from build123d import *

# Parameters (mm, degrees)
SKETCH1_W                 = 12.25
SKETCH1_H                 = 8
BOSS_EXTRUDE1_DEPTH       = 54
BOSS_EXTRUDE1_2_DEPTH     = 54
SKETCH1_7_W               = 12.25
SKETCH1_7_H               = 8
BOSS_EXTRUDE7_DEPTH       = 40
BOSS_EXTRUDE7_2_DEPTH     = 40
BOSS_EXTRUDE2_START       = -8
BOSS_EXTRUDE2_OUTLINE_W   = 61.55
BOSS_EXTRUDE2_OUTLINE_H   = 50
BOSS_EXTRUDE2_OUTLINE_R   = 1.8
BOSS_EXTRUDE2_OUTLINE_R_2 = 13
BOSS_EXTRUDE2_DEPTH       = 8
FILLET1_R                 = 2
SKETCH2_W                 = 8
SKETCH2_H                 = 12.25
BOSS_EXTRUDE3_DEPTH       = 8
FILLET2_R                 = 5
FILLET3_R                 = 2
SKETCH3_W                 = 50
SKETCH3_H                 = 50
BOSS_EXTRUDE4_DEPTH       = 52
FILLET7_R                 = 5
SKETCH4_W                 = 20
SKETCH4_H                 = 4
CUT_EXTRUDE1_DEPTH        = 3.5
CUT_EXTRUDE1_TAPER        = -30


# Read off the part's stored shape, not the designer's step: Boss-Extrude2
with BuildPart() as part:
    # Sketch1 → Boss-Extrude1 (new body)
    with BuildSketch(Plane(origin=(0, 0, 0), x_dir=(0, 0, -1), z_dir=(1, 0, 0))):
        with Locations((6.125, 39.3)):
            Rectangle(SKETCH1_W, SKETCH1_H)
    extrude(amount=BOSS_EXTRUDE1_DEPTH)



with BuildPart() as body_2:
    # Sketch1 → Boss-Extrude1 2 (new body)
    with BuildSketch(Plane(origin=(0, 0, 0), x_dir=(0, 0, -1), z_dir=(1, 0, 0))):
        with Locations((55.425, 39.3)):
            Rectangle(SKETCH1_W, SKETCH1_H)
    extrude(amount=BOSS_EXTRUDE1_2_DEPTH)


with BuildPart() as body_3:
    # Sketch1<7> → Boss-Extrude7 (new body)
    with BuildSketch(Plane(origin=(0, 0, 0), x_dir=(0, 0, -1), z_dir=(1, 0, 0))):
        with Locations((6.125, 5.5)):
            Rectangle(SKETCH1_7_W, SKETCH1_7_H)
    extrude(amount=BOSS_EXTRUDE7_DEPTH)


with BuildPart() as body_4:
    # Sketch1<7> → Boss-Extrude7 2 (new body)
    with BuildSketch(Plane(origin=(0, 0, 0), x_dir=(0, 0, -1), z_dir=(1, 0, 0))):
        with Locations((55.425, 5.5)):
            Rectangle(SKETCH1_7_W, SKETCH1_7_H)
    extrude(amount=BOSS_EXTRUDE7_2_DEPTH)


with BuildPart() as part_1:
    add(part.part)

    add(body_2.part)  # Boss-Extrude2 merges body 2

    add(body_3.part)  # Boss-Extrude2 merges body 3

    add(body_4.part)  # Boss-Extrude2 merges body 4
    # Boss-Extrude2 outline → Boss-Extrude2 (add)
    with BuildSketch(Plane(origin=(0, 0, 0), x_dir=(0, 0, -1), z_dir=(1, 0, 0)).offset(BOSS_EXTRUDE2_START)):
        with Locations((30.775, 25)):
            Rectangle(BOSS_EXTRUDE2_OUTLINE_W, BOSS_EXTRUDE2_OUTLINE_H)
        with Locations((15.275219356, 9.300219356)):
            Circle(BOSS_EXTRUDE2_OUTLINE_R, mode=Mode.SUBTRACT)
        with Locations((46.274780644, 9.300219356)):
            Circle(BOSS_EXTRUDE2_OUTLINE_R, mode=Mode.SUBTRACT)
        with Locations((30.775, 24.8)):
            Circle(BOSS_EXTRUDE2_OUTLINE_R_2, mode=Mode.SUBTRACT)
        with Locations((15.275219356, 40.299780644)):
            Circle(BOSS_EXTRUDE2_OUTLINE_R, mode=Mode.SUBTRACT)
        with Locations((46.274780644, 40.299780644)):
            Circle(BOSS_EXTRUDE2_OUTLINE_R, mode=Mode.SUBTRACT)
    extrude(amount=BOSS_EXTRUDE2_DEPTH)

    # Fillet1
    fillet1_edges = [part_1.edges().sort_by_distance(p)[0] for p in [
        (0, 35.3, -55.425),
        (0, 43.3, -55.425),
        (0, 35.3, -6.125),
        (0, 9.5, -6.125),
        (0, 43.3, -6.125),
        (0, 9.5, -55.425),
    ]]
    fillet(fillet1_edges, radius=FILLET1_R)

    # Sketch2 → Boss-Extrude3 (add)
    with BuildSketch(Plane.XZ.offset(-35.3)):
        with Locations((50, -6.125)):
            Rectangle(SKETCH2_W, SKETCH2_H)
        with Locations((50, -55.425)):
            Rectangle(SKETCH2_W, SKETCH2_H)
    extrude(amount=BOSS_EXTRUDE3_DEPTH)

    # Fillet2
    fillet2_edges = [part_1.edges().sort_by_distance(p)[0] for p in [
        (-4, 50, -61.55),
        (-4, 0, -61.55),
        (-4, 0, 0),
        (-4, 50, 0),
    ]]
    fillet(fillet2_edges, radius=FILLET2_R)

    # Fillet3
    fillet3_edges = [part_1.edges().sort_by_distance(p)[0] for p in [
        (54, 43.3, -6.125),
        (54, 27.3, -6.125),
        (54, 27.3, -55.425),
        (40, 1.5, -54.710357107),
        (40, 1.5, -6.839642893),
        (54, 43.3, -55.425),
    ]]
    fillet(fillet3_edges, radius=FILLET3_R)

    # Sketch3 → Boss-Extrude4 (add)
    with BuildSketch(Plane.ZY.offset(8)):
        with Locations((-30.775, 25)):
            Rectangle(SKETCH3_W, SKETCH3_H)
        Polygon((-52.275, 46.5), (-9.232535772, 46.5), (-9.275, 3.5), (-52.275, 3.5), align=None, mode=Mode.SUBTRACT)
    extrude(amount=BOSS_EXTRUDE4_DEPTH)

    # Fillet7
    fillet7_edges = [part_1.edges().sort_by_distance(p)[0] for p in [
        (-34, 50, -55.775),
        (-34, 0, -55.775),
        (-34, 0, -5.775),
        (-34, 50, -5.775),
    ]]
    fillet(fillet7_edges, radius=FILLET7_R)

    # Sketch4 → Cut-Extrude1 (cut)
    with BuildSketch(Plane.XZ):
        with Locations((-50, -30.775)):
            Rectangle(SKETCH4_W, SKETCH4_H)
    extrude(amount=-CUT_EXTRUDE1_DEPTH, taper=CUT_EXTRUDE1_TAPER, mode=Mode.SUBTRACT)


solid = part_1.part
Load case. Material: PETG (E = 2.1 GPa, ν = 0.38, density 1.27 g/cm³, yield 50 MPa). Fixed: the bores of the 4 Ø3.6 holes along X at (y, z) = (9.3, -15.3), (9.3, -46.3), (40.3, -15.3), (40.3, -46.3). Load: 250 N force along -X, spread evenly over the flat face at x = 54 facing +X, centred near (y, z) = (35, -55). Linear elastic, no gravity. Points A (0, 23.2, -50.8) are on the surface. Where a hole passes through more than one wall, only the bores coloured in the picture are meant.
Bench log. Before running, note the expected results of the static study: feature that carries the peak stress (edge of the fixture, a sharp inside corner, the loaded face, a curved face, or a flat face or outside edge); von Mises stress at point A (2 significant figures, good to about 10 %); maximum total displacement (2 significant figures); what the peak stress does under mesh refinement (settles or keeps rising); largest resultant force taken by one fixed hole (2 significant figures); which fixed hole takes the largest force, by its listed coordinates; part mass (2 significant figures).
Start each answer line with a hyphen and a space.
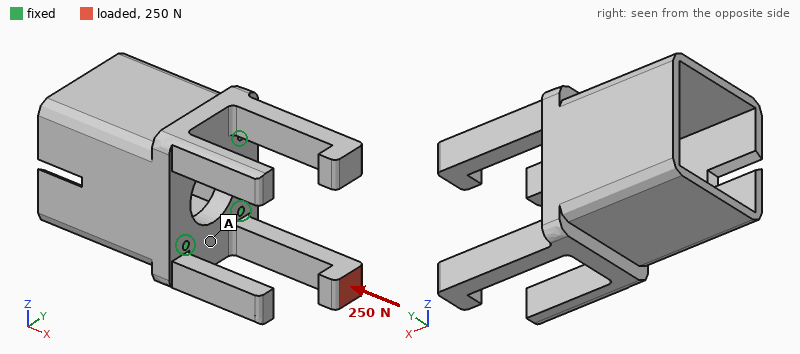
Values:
- edge of the fixture
- 1.2 MPa
- 1.6 mm
- keeps rising
- 230 N
- (40.3, -46.3)
- 91 g
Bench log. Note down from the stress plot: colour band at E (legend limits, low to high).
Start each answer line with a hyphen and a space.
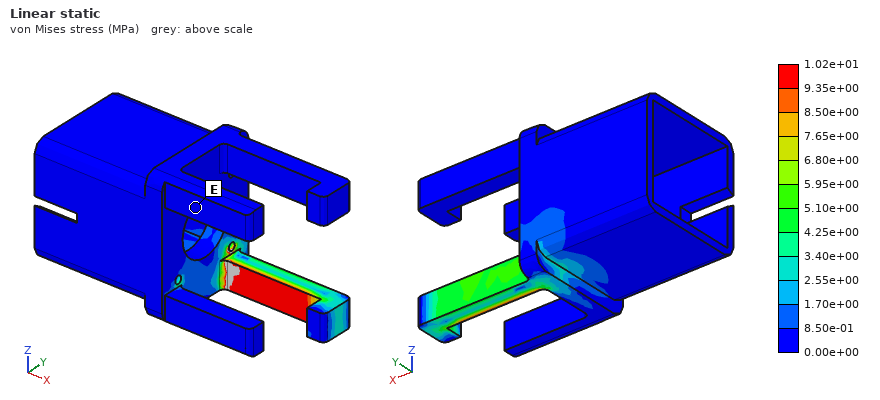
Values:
- 0.00e+00 to 8.50e-01 MPa
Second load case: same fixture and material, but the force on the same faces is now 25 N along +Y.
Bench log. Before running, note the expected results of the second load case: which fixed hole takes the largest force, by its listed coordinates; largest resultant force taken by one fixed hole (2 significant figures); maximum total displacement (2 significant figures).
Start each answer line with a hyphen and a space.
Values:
- (40.3, -46.3)
- 40 N
- 1.4 mm
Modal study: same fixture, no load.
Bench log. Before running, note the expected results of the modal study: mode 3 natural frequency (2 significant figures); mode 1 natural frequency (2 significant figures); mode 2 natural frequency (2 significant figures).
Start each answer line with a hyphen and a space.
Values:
- 530 Hz
- 420 Hz
- 420 Hz
